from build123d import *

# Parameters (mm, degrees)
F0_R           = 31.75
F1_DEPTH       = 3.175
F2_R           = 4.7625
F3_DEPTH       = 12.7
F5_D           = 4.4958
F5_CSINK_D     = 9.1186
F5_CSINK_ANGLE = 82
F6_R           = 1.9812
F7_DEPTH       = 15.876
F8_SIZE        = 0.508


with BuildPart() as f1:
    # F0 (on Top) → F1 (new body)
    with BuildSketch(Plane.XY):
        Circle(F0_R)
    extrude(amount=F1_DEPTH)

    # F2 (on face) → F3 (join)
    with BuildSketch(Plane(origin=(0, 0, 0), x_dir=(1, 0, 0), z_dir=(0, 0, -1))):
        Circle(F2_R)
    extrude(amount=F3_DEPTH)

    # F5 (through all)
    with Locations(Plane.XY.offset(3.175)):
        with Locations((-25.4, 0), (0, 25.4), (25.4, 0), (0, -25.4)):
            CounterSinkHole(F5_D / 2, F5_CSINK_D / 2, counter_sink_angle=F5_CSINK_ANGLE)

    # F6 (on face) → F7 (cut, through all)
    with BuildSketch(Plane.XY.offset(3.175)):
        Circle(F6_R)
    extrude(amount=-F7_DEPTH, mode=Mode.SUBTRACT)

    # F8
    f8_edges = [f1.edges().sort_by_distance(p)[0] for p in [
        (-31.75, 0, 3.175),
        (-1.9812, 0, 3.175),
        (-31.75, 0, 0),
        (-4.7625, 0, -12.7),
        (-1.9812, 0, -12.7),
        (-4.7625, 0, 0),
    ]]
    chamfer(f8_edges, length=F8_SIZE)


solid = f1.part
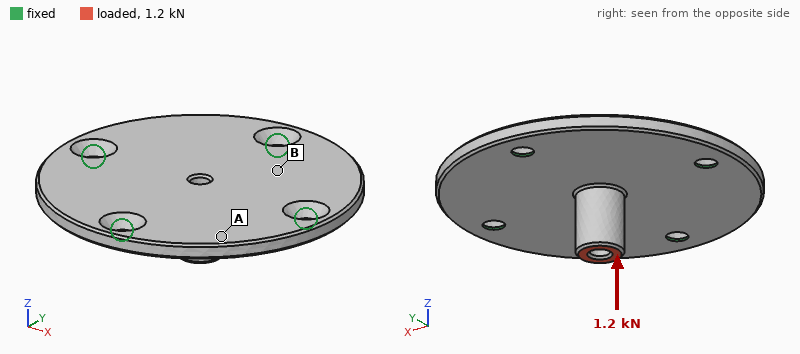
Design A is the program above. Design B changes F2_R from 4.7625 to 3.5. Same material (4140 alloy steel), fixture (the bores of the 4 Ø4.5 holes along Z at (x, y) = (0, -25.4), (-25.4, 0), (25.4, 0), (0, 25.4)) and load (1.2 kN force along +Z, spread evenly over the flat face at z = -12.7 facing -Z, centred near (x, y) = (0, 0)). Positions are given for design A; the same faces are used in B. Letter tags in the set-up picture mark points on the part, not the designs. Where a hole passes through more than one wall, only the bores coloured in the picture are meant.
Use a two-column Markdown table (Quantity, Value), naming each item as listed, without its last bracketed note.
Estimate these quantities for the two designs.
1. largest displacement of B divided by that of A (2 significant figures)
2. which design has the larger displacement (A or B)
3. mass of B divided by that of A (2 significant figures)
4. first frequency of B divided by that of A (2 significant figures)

| Quantity | Value |
|---|---|
| largest displacement of B divided by that of A | 1.2 |
| which design has the larger displacement | B |
| mass of B divided by that of A | 0.96 |
| first frequency of B divided by that of A | 1.0 |
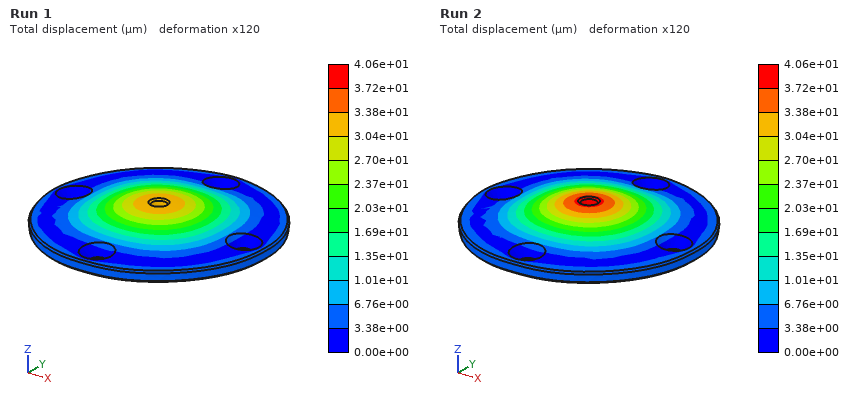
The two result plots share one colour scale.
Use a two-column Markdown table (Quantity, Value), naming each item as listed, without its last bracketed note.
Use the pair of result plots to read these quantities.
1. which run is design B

| Quantity | Value |
|---|---|
| which run is design B | Run 2 |
